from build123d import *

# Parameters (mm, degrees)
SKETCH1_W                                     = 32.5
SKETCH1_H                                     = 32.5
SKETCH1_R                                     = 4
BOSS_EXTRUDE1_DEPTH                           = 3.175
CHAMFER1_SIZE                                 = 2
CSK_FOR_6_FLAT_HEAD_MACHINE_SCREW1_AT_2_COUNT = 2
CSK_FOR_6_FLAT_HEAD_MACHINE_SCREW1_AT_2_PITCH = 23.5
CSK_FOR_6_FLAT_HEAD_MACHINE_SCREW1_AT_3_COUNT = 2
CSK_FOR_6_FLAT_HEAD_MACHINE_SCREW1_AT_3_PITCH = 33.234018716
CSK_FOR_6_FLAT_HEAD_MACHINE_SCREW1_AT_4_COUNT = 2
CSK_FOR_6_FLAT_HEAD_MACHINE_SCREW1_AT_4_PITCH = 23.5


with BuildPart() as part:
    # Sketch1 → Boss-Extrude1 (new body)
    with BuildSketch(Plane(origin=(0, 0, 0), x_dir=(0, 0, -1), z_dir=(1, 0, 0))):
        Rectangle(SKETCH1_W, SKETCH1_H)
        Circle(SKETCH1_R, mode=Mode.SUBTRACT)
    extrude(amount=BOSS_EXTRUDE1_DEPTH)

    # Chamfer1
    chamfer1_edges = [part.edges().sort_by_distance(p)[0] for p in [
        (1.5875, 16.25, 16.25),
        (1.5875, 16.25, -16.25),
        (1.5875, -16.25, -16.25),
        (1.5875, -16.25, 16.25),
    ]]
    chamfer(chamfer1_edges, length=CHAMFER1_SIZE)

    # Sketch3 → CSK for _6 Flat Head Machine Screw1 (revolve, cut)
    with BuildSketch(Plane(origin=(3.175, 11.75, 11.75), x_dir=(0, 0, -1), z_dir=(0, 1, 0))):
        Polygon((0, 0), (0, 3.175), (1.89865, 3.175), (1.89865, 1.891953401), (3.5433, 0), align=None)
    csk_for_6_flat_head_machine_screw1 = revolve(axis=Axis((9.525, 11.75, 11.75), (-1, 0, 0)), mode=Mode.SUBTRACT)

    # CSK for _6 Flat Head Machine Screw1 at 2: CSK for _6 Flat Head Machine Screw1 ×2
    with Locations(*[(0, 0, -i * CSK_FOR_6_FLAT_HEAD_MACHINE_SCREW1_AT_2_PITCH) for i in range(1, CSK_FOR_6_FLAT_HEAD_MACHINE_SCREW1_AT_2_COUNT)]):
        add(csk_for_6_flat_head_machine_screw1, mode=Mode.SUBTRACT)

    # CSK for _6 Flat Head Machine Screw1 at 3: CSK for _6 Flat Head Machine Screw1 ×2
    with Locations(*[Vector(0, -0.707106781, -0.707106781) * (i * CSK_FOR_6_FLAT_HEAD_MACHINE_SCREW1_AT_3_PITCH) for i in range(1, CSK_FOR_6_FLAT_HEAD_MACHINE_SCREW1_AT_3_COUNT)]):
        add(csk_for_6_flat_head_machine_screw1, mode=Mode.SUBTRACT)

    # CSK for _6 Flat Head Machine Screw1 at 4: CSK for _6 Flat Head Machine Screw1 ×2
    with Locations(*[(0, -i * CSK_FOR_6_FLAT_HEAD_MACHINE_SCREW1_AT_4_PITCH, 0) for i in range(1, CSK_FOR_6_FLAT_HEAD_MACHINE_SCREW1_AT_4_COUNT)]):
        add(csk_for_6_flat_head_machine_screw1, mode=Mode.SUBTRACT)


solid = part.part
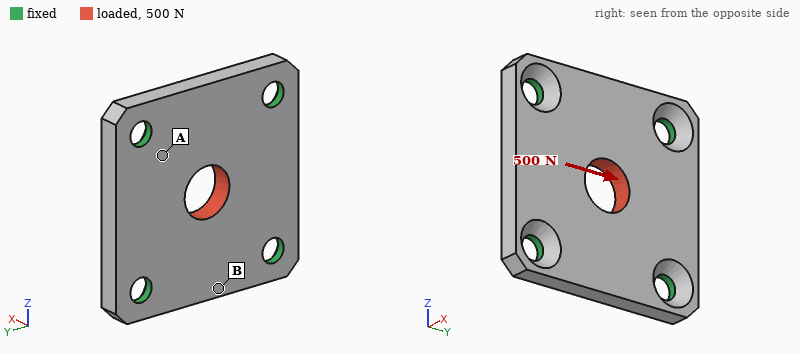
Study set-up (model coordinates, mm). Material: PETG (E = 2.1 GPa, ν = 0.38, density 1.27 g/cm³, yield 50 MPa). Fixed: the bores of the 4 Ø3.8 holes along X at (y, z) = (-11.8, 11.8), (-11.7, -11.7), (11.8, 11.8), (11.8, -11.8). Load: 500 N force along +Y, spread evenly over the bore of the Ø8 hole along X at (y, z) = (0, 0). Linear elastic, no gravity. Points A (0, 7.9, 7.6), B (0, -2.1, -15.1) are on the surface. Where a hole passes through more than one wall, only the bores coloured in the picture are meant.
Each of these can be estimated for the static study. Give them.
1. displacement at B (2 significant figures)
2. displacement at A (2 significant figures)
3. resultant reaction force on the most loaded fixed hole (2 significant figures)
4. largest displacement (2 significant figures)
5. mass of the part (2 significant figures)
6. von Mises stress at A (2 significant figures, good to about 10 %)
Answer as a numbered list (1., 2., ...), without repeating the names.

1. 11 µm
2. 22 µm
3. 140 N
4. 52 µm
5. 3.7 g
6. 7.1 MPa
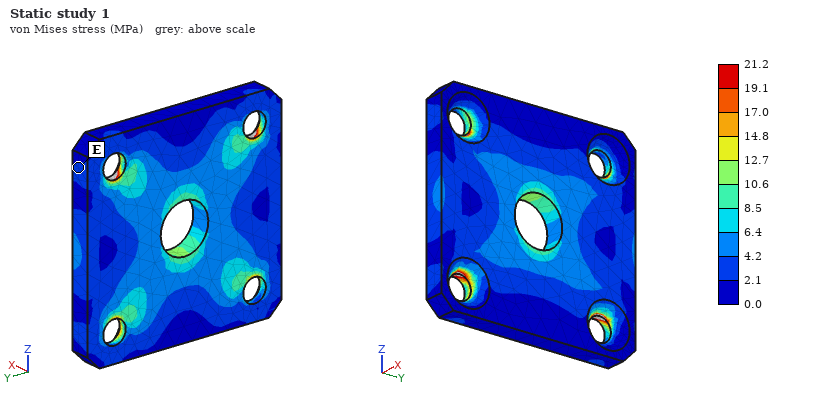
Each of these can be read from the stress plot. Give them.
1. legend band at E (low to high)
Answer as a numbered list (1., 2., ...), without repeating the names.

1. 2.1 to 4.2 MPa
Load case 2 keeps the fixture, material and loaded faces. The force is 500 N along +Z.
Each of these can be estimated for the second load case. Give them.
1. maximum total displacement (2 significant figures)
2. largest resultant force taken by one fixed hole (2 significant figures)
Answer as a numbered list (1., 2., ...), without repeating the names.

1. 52 µm
2. 140 N
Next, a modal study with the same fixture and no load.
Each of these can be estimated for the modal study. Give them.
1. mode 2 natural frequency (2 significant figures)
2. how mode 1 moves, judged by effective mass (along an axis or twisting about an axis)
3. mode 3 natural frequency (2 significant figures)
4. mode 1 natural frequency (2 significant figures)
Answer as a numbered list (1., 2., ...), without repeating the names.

1. 6600 Hz
2. along X
3. 6800 Hz
4. 4800 Hz
